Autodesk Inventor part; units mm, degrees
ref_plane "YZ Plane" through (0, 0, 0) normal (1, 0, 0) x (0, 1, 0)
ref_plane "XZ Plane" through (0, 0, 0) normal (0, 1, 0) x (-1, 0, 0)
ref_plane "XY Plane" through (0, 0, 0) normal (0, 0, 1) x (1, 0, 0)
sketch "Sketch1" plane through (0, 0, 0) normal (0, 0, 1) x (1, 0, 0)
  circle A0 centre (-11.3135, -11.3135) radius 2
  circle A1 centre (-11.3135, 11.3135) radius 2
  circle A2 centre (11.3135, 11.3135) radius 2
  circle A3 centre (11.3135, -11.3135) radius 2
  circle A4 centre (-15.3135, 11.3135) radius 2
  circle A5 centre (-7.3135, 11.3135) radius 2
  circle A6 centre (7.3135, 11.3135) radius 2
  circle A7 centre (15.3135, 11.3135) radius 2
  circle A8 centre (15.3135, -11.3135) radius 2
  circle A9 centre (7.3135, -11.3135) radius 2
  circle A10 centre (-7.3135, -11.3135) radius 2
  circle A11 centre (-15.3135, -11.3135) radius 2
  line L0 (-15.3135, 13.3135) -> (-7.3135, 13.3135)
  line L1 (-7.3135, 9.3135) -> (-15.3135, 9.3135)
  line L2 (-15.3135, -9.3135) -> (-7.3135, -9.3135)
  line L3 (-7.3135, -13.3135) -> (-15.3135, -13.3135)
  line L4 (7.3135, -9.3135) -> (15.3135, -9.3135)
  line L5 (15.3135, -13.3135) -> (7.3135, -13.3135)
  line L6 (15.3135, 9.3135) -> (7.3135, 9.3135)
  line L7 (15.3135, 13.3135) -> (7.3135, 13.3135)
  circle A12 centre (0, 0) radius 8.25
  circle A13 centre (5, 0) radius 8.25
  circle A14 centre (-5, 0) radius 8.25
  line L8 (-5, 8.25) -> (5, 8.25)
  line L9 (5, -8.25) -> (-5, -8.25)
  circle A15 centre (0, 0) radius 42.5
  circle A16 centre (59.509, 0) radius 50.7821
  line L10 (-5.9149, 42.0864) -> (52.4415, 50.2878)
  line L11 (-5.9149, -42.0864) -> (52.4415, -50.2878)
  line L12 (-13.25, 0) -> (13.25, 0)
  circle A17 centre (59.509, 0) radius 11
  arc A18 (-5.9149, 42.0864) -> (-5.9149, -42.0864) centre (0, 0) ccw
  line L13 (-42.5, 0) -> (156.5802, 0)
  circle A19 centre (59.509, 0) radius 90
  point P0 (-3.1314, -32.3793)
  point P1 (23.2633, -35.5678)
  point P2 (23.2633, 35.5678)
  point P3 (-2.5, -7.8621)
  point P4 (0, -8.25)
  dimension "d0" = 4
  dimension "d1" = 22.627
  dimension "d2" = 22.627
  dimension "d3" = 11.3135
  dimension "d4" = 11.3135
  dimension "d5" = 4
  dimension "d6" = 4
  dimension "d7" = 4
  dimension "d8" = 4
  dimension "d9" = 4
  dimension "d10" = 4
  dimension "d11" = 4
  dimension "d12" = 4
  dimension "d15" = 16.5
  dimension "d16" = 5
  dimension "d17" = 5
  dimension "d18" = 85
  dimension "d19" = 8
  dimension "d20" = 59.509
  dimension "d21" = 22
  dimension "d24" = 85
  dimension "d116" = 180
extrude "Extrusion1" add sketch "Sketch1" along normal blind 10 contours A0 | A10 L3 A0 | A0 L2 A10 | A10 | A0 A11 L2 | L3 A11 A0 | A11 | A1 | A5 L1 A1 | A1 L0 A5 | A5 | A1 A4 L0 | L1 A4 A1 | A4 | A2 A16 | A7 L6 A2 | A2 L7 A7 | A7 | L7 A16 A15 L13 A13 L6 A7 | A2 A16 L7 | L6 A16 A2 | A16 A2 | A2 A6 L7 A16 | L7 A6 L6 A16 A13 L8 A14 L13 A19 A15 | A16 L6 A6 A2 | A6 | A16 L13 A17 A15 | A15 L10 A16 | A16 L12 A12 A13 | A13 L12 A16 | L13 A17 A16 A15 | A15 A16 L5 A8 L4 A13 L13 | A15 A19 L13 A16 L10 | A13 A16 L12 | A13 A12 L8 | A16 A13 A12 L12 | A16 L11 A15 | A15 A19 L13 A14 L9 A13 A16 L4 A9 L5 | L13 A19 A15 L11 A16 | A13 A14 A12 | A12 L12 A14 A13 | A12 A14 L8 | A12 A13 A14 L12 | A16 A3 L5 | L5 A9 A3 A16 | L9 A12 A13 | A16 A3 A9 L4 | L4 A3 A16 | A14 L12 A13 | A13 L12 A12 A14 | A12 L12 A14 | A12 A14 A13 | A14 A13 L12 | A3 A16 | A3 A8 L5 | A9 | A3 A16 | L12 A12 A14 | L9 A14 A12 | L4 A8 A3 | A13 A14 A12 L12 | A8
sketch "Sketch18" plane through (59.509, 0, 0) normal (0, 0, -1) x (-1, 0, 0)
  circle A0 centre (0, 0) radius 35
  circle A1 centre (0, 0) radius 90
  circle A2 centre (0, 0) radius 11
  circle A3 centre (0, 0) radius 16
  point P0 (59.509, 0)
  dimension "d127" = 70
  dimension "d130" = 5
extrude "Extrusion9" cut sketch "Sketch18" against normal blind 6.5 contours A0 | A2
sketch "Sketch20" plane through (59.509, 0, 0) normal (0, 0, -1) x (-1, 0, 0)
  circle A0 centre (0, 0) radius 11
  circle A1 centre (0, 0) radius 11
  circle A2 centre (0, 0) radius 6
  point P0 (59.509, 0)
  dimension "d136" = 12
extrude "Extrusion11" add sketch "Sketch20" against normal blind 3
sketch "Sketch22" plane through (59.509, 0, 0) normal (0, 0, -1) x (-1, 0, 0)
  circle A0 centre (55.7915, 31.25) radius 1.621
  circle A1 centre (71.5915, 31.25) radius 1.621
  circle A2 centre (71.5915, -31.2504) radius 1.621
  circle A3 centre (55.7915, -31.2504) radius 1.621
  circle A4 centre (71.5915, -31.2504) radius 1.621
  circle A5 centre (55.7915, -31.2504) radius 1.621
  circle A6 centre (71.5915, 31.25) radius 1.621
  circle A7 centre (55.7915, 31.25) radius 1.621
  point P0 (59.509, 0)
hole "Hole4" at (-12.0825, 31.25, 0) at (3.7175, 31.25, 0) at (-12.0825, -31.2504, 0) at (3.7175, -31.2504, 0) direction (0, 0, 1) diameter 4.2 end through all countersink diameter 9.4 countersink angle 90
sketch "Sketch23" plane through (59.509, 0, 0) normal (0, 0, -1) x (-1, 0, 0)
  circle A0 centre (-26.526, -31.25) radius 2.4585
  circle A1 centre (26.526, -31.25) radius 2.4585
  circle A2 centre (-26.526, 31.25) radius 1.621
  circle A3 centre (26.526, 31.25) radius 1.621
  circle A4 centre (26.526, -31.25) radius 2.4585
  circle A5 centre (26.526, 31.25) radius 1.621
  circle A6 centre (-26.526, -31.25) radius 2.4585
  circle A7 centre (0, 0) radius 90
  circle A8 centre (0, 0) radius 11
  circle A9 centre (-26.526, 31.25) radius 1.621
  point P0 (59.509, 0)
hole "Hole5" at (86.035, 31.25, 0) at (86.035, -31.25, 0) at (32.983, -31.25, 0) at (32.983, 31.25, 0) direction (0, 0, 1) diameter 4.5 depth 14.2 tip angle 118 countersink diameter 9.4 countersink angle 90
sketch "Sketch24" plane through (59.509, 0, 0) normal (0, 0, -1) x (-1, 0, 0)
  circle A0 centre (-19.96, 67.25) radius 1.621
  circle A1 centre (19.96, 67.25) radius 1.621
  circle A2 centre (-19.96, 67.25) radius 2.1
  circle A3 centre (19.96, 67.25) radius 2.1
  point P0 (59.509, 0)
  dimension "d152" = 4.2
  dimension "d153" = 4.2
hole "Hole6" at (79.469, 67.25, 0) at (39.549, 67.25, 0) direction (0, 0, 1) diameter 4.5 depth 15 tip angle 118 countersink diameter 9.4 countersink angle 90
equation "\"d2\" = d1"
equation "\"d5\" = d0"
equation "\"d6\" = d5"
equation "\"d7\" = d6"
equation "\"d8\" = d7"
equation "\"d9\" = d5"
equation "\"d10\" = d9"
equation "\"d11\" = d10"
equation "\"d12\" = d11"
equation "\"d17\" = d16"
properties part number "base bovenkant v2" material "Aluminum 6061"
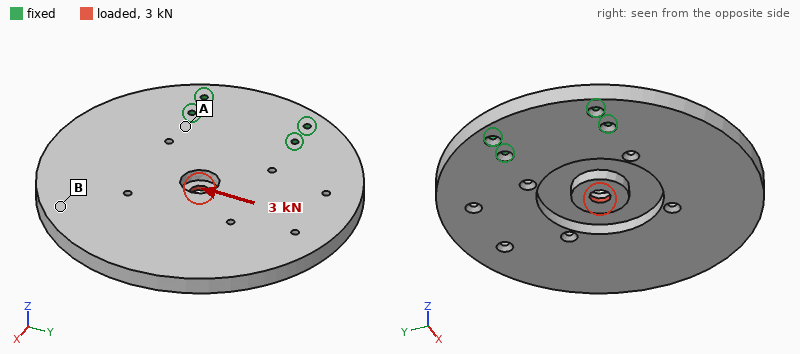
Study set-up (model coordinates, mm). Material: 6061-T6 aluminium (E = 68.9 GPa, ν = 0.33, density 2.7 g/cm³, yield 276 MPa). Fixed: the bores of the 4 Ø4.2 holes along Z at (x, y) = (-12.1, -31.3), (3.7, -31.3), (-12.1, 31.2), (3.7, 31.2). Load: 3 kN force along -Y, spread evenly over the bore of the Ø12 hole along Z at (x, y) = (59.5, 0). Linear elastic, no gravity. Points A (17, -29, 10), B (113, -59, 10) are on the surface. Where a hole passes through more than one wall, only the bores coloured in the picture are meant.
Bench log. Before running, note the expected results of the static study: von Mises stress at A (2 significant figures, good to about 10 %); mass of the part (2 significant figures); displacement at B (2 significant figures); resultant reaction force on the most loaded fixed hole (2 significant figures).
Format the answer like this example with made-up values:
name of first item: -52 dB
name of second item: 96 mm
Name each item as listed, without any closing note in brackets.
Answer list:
von Mises stress at A: 12 MPa
mass of the part: 620 g
displacement at B: 43 µm
resultant reaction force on the most loaded fixed hole: 2.4 kN
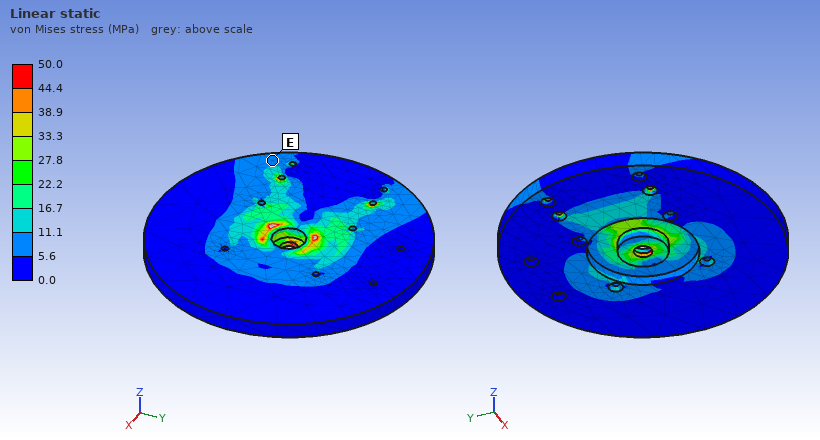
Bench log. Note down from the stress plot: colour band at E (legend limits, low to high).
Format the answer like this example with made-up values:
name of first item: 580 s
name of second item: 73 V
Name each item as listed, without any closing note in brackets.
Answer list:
colour band at E: 5.6 to 11.1 MPa
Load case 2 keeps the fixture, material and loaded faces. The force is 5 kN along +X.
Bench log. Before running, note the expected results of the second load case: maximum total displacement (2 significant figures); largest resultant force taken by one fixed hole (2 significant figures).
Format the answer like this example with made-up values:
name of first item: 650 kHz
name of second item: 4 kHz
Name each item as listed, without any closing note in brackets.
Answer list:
maximum total displacement: 0.29 mm
largest resultant force taken by one fixed hole: 1.6 kN
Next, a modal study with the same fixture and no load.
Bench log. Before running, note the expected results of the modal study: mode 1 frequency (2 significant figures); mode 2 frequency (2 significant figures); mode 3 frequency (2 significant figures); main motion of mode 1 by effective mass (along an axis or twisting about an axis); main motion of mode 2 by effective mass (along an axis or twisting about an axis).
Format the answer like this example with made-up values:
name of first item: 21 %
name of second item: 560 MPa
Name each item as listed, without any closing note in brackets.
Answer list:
mode 1 frequency: 360 Hz
mode 2 frequency: 750 Hz
mode 3 frequency: 1600 Hz
main motion of mode 1 by effective mass: along Z
main motion of mode 2 by effective mass: twisting about X
